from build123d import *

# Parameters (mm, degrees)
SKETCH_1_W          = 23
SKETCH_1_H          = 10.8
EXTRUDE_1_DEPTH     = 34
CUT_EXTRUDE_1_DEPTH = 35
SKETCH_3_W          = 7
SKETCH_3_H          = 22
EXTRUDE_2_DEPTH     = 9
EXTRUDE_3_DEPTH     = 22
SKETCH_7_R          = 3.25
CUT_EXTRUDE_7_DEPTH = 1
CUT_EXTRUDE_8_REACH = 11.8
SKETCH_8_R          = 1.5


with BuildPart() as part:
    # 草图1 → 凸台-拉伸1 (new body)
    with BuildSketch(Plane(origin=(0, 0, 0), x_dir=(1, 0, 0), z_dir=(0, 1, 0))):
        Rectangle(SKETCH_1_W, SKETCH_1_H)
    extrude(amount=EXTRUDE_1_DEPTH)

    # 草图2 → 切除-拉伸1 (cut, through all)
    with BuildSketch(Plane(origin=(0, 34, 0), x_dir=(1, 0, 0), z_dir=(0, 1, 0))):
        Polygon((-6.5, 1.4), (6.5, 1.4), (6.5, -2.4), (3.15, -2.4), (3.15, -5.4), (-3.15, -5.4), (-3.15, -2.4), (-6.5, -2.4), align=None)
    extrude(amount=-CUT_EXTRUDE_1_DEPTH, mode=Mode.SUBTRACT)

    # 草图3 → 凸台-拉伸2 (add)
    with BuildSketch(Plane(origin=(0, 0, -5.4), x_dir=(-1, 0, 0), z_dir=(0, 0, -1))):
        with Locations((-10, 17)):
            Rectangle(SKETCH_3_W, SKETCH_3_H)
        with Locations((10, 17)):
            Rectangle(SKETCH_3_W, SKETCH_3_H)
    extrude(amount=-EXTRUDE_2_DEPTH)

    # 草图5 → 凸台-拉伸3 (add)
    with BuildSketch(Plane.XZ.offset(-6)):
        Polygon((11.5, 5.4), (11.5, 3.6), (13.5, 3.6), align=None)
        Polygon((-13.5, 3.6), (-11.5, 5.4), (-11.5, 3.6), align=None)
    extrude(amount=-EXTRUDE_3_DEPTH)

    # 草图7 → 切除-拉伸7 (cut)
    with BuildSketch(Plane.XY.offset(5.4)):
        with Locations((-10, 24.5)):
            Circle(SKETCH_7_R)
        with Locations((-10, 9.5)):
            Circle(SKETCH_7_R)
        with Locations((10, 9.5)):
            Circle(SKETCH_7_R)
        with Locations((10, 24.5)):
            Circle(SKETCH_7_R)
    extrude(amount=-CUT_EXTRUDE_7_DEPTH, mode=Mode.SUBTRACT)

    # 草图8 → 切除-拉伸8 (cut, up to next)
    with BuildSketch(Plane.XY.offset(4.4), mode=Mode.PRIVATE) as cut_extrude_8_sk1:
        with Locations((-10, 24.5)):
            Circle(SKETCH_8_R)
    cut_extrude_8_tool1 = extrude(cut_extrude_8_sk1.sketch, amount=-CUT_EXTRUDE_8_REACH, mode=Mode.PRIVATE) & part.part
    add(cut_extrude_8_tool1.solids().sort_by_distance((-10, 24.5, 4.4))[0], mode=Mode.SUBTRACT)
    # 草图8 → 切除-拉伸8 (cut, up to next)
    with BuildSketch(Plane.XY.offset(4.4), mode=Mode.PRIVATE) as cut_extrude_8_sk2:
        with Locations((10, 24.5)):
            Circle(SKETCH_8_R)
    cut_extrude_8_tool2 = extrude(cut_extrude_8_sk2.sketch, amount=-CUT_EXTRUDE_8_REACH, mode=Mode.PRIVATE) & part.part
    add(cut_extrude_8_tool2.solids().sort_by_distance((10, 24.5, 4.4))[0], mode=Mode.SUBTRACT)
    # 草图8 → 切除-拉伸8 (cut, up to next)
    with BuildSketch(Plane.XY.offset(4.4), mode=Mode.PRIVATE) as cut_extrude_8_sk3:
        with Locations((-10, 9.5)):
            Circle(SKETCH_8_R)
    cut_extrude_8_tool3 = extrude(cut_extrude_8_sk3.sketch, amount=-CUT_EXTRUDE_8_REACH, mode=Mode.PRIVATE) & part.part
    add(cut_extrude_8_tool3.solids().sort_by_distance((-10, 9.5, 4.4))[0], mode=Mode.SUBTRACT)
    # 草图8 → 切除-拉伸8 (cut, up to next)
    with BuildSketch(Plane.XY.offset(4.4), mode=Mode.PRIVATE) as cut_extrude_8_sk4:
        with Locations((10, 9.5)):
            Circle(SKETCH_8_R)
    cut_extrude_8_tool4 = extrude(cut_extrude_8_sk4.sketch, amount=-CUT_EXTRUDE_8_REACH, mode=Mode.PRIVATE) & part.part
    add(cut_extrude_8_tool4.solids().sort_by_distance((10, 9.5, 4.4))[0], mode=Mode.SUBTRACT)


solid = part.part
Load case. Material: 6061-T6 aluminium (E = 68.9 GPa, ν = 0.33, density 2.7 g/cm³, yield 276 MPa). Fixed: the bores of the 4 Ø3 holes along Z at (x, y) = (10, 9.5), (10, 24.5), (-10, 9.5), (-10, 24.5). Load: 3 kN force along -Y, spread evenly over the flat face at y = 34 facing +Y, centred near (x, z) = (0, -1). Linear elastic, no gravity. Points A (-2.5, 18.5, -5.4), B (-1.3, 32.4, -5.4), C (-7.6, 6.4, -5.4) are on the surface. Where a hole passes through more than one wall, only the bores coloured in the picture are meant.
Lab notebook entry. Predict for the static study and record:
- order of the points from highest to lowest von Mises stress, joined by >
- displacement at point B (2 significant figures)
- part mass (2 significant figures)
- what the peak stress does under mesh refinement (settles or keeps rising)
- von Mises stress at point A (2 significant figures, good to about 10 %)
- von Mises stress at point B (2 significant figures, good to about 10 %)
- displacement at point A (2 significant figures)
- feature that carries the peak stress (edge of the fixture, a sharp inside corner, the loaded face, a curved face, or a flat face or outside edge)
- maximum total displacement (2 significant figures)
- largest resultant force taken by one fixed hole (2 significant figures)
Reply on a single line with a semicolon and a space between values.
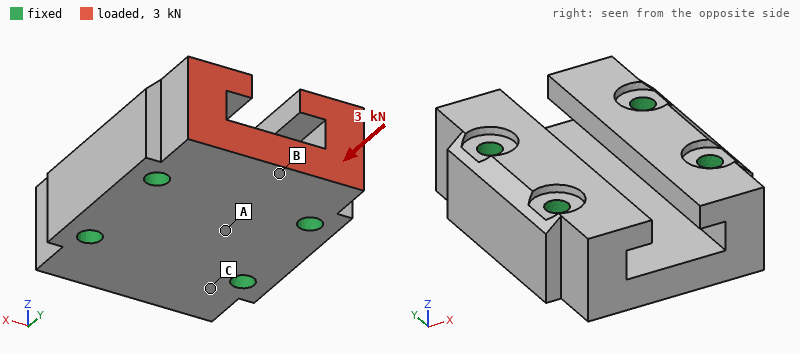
B > A > C; 3.4 µm; 18 g; keeps rising; 7.8 MPa; 14 MPa; 0.99 µm; edge of the fixture; 4.5 µm; 1.3 kN
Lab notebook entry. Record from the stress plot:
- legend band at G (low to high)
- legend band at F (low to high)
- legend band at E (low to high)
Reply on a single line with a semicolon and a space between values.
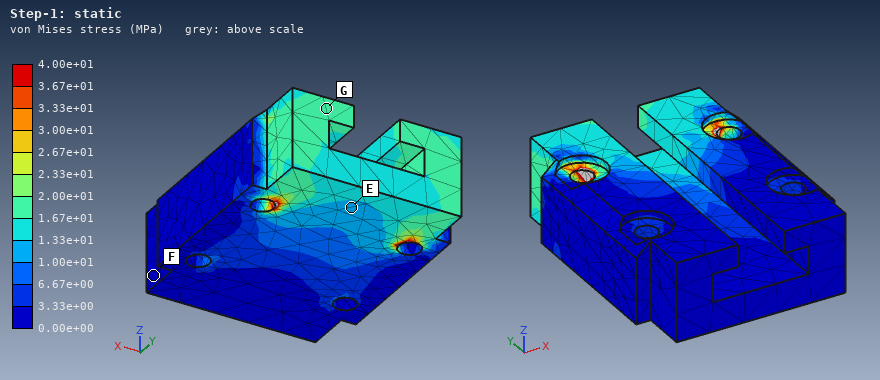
1.67e+01 to 2.00e+01 MPa; 0.00e+00 to 3.33e+00 MPa; 1.00e+01 to 1.33e+01 MPa
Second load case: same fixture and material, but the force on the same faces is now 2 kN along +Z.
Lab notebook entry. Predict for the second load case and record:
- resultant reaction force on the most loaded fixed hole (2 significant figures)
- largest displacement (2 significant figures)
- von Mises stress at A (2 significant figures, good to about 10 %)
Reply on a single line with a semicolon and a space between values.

1.1 kN; 23 µm; 12 MPa
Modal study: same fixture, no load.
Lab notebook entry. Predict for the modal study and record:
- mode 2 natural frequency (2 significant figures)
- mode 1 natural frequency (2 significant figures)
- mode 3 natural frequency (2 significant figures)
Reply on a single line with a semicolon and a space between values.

42 kHz; 42 kHz; 53 kHz
